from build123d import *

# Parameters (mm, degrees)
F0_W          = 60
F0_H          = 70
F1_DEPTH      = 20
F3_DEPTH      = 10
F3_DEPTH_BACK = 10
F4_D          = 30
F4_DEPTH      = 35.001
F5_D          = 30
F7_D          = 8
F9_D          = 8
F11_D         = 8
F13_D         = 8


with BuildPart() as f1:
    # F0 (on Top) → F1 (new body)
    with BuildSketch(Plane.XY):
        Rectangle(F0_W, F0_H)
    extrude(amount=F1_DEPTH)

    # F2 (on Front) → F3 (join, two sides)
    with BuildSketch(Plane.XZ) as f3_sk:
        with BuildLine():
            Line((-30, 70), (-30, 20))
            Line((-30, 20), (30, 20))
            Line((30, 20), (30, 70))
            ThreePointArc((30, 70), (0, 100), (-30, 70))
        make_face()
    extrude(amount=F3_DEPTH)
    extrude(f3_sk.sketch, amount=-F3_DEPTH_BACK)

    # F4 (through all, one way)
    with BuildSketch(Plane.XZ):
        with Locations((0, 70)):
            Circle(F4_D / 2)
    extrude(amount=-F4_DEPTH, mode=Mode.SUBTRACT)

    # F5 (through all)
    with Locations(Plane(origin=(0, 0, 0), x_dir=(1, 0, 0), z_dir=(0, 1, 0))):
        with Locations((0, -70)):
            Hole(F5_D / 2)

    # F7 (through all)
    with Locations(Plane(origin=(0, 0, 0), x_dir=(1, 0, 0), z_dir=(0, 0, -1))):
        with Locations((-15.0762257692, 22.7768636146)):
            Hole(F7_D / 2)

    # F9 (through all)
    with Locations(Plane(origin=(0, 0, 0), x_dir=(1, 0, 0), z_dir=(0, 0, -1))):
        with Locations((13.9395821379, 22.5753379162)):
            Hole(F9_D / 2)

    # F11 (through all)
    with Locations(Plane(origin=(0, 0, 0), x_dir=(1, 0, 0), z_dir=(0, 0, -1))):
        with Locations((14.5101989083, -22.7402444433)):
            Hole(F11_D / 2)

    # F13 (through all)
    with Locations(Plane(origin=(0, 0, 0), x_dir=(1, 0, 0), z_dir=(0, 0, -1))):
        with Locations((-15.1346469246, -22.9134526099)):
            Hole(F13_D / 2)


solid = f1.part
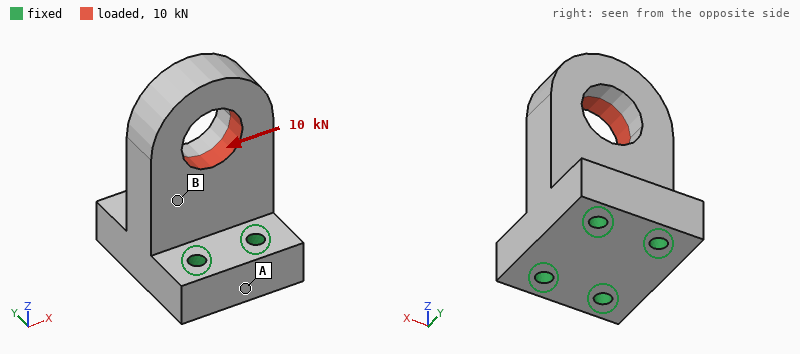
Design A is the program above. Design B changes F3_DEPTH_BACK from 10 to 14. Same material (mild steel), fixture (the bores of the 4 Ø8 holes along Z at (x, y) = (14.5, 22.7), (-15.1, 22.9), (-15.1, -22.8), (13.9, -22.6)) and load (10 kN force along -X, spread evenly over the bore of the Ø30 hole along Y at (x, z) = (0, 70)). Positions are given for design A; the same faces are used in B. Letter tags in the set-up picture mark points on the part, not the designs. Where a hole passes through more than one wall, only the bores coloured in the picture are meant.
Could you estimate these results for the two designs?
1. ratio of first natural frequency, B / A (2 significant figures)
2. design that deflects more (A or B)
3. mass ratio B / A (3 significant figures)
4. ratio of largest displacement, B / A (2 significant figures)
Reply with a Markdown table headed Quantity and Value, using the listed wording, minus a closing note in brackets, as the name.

| Quantity | Value |
|---|---|
| ratio of first natural frequency, B / A | 1.1 |
| design that deflects more | A |
| mass ratio B / A | 1.10 |
| ratio of largest displacement, B / A | 0.86 |
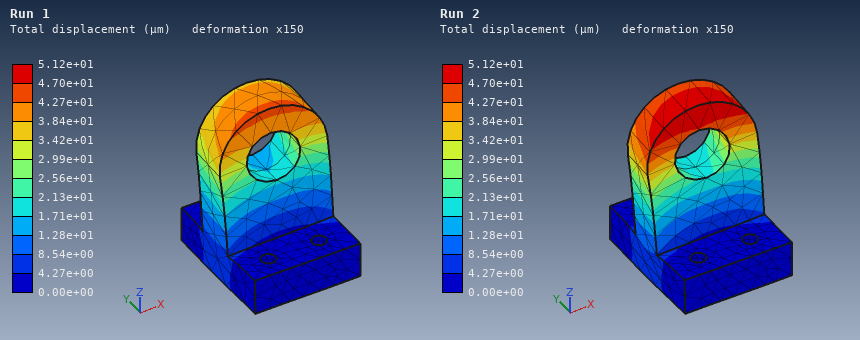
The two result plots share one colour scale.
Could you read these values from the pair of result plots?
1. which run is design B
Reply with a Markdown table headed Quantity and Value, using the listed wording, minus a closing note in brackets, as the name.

| Quantity | Value |
|---|---|
| which run is design B | Run 1 |
